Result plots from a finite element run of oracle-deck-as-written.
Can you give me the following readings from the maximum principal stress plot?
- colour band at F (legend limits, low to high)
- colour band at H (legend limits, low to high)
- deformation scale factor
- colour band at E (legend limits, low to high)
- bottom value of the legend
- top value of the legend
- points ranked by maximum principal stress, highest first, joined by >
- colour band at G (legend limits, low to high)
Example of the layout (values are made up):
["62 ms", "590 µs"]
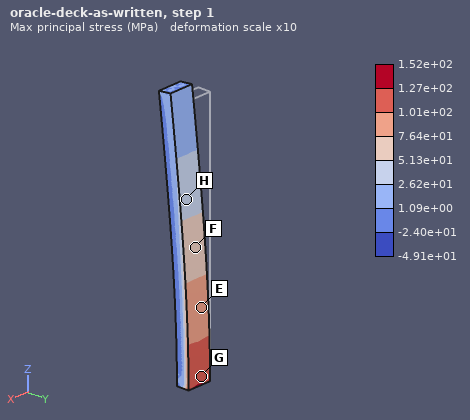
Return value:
["5.13e+01 to 7.64e+01 MPa", "2.62e+01 to 5.13e+01 MPa", "10", "7.64e+01 to 1.01e+02 MPa", "-4.91e+01 MPa", "1.52e+02 MPa", "G > E > F > H", "1.01e+02 to 1.27e+02 MPa"]
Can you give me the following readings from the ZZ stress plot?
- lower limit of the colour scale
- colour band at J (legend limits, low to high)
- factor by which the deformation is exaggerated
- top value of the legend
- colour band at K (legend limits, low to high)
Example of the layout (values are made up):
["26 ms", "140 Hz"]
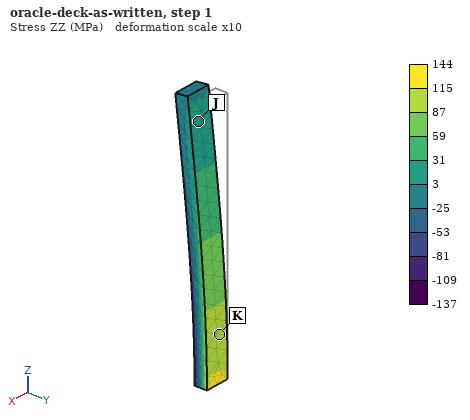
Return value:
["-137 MPa", "3 to 31 MPa", "10", "144 MPa", "87 to 115 MPa"]
